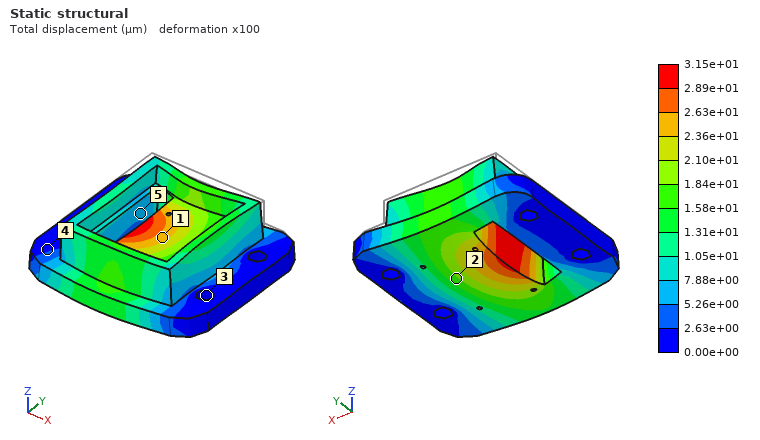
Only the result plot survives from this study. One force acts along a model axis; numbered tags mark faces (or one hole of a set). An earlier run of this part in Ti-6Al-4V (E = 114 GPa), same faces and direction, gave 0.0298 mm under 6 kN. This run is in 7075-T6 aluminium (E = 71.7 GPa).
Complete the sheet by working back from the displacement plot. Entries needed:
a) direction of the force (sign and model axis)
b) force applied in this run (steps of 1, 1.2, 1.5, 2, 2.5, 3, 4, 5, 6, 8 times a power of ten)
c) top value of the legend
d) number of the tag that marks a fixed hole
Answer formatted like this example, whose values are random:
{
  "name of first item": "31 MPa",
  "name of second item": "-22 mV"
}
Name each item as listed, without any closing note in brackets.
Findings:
{
  "direction of the force": "-Z",
  "force applied in this run": "4 kN",
  "top value of the legend": "3.15e+01 µm",
  "number of the tag that marks a fixed hole": "3"
}
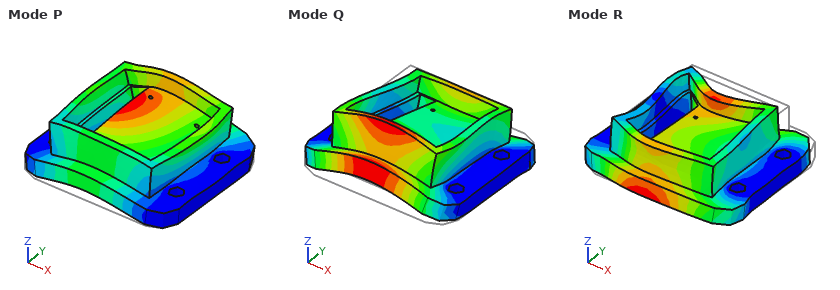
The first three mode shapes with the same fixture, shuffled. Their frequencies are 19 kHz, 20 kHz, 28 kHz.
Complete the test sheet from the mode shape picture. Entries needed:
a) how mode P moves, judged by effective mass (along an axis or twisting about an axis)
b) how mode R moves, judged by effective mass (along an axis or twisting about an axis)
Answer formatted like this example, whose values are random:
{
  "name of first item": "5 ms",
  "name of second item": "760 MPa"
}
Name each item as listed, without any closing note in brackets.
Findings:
{
  "how mode P moves, judged by effective mass": "along Z",
  "how mode R moves, judged by effective mass": "along Y"
}
